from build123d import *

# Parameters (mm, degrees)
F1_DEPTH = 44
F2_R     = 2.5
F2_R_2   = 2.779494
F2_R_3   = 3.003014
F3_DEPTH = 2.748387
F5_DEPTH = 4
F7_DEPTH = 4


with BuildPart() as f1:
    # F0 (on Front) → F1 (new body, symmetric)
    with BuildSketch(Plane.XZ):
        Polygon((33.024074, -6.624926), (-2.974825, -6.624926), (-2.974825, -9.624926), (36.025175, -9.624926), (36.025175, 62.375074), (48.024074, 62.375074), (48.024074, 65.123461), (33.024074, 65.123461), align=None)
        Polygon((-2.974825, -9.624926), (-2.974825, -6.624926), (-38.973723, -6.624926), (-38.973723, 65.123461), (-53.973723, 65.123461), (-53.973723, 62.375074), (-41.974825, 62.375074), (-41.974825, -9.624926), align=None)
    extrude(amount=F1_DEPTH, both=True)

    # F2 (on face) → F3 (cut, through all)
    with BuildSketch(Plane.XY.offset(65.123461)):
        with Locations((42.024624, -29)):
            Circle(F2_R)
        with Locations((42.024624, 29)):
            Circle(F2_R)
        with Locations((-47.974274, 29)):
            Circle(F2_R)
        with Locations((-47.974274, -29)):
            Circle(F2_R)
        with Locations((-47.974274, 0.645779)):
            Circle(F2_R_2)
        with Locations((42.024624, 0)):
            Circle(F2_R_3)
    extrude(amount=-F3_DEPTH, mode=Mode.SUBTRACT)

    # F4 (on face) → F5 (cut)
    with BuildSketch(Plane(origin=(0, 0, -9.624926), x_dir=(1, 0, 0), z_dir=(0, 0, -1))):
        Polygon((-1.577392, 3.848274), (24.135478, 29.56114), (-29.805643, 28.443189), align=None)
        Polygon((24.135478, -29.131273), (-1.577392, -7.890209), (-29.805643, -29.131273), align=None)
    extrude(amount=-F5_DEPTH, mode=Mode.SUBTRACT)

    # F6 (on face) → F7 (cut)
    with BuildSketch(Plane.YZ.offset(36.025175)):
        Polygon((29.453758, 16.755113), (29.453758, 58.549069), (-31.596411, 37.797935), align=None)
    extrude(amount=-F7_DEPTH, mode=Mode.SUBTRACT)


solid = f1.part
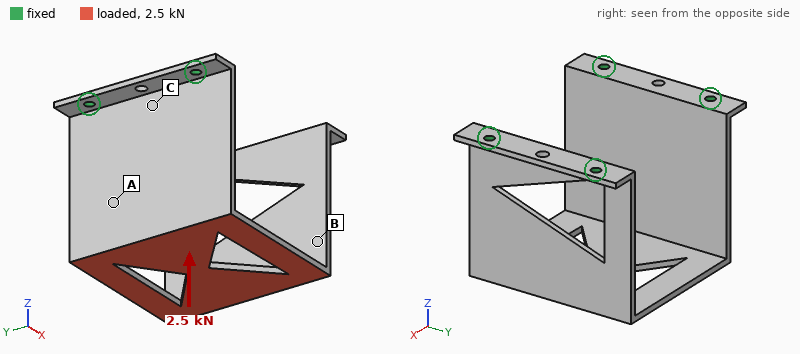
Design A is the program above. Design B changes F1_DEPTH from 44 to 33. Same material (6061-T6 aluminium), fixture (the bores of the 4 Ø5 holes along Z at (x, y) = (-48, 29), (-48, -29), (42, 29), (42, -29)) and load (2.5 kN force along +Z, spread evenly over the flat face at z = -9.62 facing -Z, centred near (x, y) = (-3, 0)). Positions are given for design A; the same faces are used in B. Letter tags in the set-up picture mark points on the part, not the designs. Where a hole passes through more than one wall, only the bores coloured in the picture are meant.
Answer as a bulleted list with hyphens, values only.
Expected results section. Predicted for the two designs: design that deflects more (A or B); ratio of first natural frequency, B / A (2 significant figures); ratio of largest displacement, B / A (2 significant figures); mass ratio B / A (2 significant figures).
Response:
- B
- 0.96
- 1.5
- 0.71
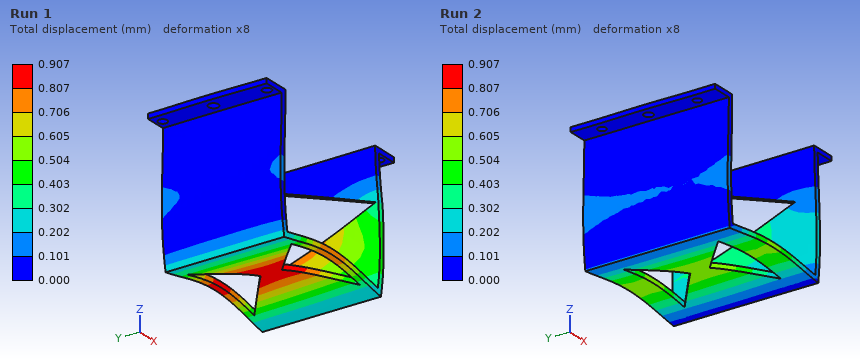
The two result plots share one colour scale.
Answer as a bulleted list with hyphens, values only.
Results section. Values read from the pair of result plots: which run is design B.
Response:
- Run 1
